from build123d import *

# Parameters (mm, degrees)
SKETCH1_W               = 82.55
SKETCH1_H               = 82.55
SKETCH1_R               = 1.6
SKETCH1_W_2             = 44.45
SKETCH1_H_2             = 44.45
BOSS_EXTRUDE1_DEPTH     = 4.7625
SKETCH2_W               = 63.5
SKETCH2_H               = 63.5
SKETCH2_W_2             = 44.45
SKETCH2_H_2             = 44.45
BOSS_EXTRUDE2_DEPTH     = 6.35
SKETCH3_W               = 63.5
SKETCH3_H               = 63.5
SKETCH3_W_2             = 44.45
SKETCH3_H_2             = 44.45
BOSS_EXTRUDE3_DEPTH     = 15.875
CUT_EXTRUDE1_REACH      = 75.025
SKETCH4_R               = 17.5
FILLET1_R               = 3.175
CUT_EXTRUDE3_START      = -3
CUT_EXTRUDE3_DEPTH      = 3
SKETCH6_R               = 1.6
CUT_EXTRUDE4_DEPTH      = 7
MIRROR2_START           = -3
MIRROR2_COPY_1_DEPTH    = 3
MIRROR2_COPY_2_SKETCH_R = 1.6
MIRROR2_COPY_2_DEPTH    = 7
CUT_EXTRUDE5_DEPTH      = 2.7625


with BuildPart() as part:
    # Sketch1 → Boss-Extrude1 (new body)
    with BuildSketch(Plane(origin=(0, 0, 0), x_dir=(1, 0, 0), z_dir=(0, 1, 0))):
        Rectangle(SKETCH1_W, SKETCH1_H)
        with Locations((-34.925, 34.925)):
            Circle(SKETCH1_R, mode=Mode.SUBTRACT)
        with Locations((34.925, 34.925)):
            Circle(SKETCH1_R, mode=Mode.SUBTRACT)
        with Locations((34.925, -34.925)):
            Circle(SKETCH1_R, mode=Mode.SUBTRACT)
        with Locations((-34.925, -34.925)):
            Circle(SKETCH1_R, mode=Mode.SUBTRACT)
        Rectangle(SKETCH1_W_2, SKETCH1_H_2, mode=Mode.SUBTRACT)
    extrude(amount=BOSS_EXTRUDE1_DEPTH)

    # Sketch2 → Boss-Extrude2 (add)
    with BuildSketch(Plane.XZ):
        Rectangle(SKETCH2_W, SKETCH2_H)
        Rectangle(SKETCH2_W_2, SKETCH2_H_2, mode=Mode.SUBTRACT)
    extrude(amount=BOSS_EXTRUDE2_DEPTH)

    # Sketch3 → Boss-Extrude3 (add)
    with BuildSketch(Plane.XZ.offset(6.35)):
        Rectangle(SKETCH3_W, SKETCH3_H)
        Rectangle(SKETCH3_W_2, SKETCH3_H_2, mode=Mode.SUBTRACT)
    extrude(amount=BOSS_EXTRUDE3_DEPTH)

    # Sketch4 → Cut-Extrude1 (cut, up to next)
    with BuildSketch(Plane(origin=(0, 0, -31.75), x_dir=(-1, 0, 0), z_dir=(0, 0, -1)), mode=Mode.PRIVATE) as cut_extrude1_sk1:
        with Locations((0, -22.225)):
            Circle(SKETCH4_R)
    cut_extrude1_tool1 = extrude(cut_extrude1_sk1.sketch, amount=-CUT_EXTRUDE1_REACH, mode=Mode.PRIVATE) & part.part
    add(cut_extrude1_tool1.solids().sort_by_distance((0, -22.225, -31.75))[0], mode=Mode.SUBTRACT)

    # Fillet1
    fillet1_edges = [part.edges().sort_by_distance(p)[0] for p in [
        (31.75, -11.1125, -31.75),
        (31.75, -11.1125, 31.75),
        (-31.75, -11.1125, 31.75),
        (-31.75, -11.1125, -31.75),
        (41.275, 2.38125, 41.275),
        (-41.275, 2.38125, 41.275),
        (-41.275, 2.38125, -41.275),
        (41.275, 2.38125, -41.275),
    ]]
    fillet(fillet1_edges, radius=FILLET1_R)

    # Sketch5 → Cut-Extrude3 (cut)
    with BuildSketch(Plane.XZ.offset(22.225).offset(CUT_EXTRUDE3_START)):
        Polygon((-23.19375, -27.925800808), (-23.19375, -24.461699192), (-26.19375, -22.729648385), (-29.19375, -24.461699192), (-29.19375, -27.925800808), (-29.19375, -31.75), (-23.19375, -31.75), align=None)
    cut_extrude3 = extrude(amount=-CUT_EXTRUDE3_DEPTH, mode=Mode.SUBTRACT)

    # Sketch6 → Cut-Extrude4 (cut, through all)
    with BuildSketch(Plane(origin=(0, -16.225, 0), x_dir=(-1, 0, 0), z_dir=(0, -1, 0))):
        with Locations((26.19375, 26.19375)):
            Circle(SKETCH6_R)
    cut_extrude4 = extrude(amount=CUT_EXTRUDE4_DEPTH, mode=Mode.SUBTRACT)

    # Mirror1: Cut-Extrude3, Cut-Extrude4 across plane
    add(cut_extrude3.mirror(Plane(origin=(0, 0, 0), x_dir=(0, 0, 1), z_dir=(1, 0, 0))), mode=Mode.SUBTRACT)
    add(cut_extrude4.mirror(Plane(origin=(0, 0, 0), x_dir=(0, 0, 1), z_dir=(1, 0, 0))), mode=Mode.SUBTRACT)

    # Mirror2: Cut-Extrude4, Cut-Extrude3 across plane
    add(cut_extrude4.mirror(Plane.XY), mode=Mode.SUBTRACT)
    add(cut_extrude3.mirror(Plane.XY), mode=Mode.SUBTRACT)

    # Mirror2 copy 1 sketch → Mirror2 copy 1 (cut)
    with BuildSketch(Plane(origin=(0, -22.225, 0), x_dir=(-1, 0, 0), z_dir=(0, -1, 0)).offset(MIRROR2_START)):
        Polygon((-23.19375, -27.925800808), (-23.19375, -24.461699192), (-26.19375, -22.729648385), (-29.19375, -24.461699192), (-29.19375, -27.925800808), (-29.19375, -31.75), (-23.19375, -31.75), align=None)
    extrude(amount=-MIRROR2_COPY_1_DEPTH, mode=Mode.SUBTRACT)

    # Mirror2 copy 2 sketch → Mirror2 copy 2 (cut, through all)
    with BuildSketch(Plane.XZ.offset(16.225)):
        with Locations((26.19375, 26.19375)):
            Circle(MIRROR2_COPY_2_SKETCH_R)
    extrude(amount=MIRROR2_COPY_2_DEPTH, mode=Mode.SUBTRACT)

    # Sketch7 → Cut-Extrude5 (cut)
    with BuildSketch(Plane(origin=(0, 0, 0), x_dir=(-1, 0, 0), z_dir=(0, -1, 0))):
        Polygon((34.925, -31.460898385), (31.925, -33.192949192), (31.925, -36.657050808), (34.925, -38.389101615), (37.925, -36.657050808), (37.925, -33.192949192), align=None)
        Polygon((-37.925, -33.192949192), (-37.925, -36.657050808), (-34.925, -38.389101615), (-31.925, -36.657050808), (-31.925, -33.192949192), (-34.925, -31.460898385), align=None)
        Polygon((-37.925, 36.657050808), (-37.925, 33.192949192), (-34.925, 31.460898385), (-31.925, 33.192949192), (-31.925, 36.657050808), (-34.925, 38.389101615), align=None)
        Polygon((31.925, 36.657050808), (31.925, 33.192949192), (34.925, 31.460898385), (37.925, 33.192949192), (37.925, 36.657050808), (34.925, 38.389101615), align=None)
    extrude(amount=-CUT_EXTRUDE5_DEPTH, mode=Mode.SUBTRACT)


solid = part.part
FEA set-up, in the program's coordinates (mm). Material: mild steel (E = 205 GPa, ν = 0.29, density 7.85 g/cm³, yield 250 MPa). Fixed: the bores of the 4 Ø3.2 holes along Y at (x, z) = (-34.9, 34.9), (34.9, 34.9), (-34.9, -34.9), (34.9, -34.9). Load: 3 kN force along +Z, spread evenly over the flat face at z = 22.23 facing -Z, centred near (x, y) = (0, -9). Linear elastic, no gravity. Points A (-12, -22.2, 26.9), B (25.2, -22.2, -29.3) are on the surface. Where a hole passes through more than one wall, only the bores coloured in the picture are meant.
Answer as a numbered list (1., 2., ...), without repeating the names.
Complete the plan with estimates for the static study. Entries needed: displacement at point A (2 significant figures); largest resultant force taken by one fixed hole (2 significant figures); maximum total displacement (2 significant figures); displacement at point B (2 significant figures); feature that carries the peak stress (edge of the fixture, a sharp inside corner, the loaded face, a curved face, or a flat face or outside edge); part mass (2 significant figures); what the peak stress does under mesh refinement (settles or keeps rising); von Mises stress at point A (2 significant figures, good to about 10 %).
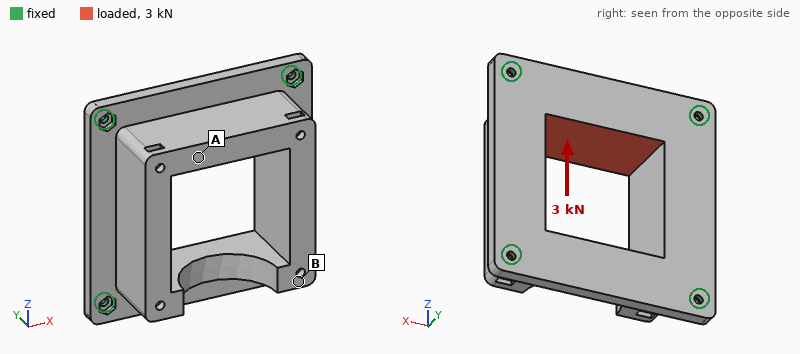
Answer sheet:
1. 8.0 µm
2. 880 N
3. 9.9 µm
4. 2.4 µm
5. edge of the fixture
6. 490 g
7. keeps rising
8. 13 MPa
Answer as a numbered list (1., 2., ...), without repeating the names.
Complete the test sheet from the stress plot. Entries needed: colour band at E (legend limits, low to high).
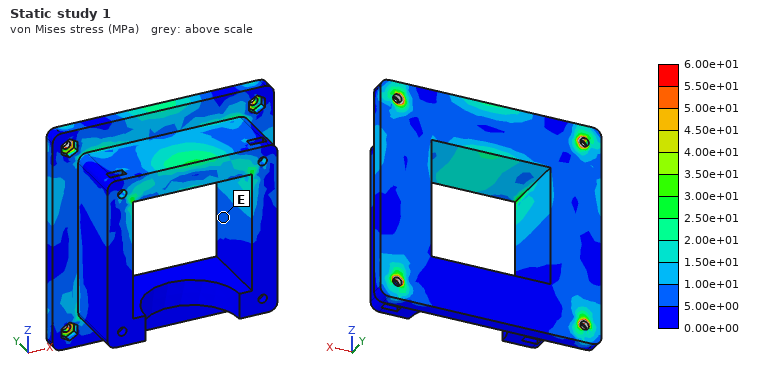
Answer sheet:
1. 5.00e+00 to 1.00e+01 MPa
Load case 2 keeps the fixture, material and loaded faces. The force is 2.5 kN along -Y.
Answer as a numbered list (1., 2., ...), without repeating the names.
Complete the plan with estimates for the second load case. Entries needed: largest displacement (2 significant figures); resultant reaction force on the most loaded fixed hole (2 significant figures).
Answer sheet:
1. 10 µm
2. 1.4 kN
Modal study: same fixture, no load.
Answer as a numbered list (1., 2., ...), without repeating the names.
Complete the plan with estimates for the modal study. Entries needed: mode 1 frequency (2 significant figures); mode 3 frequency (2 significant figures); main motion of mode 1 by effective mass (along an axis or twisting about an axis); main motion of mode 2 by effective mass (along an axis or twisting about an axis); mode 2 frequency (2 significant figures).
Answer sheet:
1. 4600 Hz
2. 6300 Hz
3. along Y
4. along Y
5. 5800 Hz
